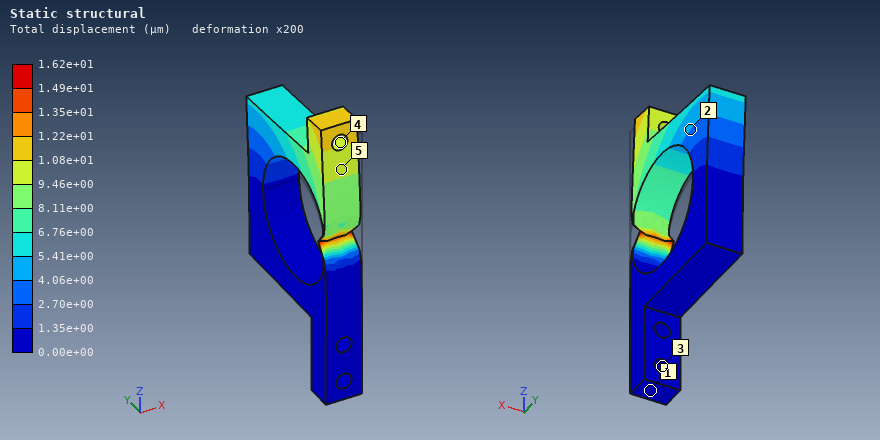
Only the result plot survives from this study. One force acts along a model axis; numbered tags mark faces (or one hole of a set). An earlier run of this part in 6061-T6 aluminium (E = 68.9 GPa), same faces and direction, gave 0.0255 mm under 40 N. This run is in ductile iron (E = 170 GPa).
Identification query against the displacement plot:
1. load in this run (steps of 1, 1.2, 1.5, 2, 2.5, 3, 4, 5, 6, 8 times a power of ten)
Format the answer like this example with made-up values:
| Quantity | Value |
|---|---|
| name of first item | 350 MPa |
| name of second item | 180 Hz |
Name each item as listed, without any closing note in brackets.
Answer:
| Quantity | Value |
|---|---|
| load in this run | 60 N |
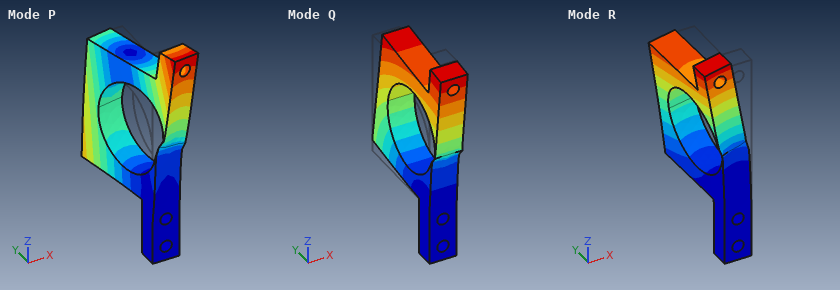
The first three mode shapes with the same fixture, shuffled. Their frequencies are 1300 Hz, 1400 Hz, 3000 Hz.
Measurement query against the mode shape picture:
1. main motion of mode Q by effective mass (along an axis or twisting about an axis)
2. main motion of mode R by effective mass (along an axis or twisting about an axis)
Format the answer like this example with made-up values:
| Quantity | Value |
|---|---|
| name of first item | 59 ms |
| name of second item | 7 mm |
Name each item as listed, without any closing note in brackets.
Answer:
| Quantity | Value |
|---|---|
| main motion of mode Q by effective mass | along Y |
| main motion of mode R by effective mass | along X |
